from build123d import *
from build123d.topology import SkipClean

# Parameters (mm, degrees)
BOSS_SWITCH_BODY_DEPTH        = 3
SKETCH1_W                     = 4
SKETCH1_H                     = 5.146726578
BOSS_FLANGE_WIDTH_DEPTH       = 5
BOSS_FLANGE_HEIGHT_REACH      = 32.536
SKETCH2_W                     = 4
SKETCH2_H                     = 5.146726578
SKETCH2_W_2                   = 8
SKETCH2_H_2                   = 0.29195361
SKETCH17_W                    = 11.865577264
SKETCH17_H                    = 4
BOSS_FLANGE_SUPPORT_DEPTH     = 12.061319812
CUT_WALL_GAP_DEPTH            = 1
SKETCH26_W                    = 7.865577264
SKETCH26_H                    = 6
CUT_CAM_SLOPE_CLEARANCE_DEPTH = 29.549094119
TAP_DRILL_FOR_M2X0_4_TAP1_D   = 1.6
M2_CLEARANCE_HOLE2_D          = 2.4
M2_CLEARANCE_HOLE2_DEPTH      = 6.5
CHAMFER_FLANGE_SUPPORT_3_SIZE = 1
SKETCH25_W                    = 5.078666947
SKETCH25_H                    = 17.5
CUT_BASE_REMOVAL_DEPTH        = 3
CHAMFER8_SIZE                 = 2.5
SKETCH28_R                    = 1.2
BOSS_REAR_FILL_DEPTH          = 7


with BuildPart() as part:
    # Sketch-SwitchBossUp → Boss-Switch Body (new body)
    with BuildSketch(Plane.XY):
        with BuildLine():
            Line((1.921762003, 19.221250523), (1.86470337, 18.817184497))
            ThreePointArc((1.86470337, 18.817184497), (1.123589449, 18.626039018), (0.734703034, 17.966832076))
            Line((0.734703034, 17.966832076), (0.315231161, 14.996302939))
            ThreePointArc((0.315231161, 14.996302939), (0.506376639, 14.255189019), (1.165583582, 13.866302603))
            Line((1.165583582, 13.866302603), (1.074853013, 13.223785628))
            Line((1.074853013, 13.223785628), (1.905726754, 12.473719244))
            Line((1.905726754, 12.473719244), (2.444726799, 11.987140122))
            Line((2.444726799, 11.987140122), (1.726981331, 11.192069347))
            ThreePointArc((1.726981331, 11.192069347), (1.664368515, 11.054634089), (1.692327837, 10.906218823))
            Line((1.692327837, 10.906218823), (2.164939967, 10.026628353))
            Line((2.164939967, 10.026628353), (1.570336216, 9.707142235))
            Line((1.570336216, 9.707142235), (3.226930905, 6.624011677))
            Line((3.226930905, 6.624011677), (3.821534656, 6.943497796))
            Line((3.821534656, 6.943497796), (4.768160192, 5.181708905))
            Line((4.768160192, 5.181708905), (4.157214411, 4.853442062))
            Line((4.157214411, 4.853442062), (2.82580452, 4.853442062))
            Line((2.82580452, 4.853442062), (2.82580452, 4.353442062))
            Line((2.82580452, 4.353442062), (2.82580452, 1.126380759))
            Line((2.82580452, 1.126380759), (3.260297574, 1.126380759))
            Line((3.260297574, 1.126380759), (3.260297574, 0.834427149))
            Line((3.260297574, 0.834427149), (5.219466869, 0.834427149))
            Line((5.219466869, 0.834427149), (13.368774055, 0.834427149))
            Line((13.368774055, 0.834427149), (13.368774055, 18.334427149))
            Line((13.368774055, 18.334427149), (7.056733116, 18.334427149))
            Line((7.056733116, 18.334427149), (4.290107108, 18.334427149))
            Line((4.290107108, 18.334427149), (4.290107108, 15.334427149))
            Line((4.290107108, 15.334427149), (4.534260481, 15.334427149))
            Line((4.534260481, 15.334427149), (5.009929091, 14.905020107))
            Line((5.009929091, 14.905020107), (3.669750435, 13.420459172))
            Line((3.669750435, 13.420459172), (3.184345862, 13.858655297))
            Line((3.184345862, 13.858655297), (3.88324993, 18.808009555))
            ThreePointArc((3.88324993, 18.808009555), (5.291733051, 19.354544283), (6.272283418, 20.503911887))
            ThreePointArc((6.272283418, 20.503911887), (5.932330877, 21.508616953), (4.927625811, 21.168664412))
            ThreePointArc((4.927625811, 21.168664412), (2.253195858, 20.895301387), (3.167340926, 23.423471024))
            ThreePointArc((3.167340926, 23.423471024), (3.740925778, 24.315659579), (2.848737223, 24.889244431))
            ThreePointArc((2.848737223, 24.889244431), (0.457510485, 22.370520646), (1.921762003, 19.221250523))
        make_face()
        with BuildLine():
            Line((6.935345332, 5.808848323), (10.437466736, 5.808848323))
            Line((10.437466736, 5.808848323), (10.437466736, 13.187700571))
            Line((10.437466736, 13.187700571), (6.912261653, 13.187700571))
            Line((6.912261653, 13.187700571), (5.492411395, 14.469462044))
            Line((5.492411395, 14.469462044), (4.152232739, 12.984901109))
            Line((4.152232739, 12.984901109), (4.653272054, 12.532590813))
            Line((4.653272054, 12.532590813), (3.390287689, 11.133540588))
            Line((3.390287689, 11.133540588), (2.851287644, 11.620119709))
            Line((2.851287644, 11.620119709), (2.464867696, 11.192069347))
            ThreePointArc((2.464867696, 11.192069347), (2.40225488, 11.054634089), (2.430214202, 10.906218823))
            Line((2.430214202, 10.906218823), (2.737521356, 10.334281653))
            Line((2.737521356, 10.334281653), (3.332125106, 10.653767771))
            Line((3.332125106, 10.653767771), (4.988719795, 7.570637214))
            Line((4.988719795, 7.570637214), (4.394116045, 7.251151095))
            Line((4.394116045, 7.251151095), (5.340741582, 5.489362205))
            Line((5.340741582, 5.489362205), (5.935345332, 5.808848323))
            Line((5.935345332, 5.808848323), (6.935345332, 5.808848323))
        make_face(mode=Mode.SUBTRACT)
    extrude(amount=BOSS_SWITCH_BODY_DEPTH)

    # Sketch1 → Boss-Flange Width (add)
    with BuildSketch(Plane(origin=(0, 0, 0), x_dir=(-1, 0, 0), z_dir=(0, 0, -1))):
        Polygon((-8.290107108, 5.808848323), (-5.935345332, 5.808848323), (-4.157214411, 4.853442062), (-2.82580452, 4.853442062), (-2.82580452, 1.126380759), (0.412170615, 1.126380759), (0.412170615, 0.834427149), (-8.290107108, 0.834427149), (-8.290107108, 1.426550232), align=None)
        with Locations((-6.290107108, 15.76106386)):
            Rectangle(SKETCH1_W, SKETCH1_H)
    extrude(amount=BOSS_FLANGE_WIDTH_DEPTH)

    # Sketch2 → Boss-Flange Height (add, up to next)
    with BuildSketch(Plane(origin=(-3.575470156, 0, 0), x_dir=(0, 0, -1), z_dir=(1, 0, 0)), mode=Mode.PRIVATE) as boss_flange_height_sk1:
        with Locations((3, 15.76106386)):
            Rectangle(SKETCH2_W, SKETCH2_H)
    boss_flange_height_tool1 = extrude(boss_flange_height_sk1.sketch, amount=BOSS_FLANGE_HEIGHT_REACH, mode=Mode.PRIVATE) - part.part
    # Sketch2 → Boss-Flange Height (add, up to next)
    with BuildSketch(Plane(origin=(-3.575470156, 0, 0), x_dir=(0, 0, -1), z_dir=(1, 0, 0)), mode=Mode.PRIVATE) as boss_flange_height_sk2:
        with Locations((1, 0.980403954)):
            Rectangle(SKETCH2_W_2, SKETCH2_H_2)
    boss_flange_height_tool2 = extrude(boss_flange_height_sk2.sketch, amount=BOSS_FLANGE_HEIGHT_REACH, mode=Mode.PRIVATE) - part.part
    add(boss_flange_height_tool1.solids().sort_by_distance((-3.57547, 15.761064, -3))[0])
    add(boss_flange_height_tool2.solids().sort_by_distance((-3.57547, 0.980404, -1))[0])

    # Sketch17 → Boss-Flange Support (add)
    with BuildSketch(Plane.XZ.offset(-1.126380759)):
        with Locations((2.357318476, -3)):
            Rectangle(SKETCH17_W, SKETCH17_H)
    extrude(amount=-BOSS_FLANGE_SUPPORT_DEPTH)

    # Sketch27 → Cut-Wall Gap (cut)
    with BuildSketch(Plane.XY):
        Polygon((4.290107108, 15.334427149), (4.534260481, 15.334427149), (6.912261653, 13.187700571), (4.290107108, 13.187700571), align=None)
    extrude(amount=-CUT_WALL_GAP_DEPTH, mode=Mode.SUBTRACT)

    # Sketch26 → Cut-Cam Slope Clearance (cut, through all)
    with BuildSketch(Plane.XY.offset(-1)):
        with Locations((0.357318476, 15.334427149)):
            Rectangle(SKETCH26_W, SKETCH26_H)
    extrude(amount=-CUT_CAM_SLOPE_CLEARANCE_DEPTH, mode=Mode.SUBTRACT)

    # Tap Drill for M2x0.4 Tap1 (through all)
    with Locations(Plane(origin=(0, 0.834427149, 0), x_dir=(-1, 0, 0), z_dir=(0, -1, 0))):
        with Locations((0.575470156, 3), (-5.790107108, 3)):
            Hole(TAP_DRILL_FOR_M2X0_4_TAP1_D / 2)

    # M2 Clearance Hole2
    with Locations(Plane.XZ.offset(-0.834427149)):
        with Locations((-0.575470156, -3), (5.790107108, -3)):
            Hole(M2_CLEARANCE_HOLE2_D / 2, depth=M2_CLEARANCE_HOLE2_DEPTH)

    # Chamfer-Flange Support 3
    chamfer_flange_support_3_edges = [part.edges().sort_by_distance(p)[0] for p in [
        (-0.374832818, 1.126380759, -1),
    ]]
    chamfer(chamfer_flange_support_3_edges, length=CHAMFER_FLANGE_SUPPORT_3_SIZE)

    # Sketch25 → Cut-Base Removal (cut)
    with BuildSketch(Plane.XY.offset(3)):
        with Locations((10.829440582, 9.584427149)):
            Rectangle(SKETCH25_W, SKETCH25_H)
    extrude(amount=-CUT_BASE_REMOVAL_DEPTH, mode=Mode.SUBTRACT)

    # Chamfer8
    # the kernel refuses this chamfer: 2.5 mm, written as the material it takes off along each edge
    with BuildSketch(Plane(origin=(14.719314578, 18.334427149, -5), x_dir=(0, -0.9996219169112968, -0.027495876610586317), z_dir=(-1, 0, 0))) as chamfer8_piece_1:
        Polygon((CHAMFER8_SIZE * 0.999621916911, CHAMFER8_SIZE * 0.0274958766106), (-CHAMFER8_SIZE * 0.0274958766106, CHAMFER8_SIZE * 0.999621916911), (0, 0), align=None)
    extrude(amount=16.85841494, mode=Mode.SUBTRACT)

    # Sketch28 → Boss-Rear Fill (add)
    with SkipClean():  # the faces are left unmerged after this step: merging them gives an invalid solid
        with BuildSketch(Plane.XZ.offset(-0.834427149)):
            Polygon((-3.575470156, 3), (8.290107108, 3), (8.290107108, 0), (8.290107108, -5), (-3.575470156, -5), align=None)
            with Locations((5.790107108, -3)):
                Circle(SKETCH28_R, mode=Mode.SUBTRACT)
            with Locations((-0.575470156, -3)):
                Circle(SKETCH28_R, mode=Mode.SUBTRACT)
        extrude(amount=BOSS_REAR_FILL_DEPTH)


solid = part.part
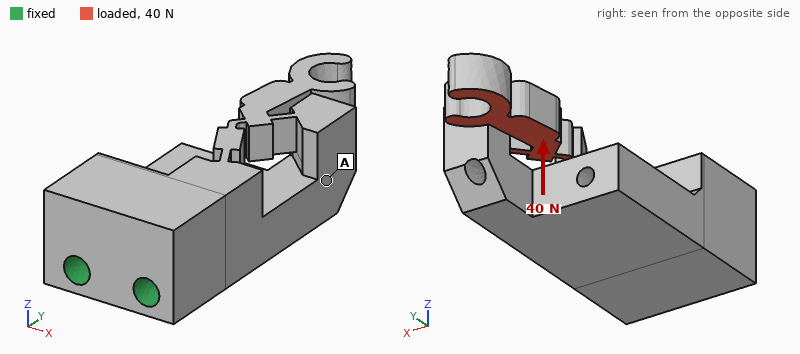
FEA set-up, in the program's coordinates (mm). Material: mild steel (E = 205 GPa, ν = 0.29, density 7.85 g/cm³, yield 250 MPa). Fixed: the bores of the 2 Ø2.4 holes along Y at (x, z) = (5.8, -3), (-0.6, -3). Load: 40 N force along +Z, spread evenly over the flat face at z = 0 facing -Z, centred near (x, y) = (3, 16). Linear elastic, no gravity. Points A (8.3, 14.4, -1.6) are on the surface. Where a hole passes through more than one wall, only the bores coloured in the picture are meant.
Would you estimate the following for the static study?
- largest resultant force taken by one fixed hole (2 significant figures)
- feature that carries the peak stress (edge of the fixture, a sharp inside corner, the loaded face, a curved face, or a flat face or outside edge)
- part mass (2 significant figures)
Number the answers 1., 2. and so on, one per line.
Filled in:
1. 25 N
2. a curved face
3. 11 g
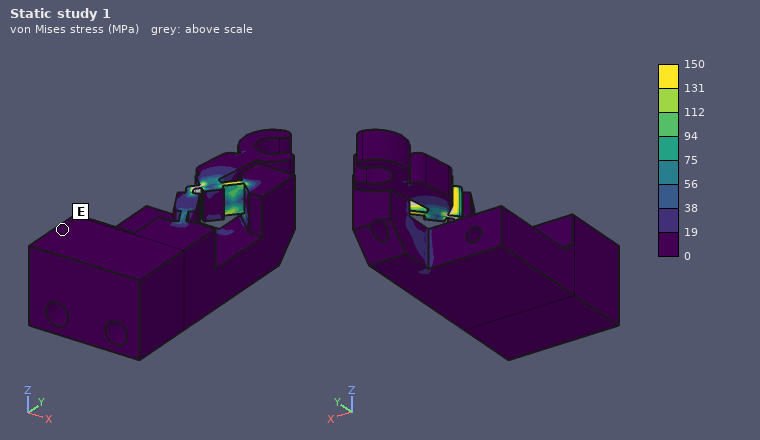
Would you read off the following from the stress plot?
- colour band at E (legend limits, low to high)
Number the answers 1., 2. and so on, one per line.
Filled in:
1. 0 to 19 MPa
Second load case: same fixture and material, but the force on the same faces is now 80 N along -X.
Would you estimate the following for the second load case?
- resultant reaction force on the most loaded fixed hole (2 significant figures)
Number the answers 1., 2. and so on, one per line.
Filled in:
1. 160 N
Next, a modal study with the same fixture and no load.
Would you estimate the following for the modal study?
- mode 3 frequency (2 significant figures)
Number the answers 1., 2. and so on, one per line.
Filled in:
1. 13 kHz
